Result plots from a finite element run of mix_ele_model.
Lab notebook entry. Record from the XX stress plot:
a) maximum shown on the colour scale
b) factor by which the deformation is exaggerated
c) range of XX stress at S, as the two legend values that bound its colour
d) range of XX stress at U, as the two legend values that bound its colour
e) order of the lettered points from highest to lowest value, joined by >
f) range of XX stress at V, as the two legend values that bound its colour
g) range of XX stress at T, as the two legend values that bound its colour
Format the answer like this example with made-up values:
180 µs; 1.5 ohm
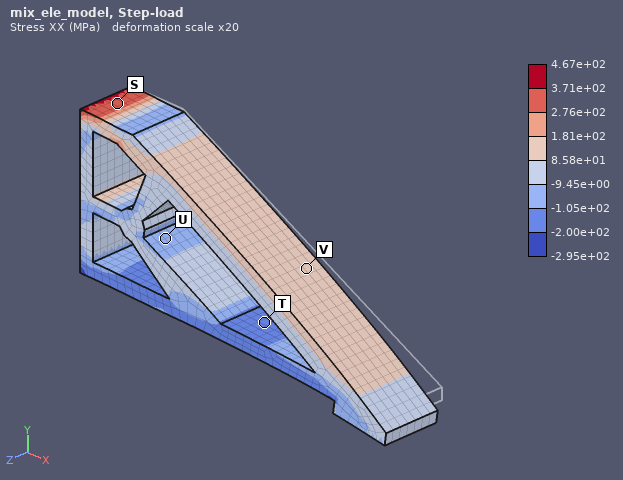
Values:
4.67e+02 MPa; 20; 2.76e+02 to 3.71e+02 MPa; -1.05e+02 to -9.45e+00 MPa; S > V > U > T; 8.58e+01 to 1.81e+02 MPa; -2.00e+02 to -1.05e+02 MPa
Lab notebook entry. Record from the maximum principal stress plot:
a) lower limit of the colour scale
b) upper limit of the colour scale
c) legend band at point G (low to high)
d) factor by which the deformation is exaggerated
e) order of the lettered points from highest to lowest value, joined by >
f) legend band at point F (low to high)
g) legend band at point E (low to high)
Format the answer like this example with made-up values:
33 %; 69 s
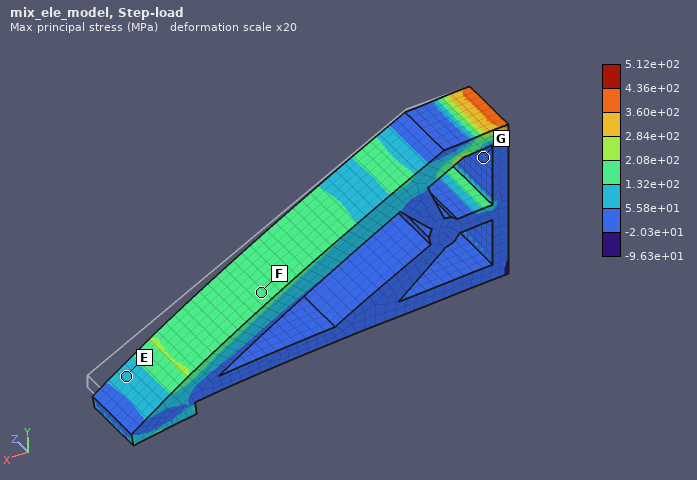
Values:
-9.63e+01 MPa; 5.12e+02 MPa; -2.03e+01 to 5.58e+01 MPa; 20; F > E > G; 1.32e+02 to 2.08e+02 MPa; 5.58e+01 to 1.32e+02 MPa
